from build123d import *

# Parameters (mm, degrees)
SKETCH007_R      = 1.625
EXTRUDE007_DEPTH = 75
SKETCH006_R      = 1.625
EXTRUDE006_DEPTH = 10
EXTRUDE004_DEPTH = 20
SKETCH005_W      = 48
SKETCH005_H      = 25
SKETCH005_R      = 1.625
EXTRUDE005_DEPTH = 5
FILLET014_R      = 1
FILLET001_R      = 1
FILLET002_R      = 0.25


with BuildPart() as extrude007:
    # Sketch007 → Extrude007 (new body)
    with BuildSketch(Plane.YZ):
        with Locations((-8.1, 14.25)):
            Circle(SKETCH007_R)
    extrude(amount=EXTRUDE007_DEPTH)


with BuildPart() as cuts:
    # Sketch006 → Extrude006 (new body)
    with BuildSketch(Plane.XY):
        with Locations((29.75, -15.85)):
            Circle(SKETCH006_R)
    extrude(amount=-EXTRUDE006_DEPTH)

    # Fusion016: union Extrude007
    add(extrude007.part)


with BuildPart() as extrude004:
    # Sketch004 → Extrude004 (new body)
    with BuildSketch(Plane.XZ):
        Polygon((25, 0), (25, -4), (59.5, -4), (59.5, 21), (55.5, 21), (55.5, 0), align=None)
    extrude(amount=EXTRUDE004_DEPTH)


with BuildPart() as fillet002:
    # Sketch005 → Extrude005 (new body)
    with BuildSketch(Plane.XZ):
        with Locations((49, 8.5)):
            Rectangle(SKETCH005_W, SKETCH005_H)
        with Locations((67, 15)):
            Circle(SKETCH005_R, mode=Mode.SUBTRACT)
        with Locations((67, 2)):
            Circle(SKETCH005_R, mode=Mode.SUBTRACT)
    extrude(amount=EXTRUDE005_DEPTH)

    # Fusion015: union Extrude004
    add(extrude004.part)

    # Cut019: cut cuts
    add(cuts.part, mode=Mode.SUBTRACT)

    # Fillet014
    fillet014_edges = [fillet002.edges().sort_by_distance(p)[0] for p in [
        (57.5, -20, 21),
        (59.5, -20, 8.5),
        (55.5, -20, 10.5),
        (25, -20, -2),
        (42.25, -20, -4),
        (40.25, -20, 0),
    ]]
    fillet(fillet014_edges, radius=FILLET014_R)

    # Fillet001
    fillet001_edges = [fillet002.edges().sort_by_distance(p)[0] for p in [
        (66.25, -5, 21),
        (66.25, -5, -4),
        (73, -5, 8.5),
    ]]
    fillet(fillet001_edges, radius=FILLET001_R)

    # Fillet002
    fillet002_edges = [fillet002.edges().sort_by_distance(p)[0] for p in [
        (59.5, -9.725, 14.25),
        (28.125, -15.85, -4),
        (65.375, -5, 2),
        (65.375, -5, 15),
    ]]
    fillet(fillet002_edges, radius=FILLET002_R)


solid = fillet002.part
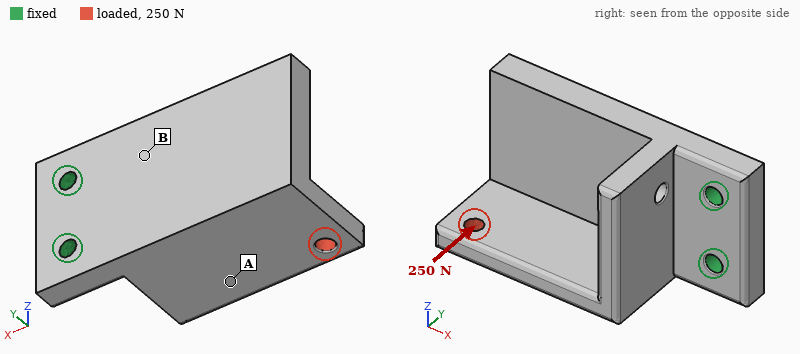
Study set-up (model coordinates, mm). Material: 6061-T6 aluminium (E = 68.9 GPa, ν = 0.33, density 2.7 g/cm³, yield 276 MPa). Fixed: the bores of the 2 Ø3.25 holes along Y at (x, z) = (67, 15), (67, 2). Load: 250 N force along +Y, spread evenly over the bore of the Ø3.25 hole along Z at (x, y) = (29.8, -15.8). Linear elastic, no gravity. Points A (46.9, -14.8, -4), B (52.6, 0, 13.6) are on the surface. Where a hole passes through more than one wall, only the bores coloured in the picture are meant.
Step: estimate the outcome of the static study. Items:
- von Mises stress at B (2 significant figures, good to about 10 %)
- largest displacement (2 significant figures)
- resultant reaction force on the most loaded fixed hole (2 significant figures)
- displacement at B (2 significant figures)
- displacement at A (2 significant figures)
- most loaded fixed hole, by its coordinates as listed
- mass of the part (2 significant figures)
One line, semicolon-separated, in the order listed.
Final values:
30 MPa; 0.24 mm; 270 N; 0.041 mm; 0.11 mm; (67, 2); 25 g
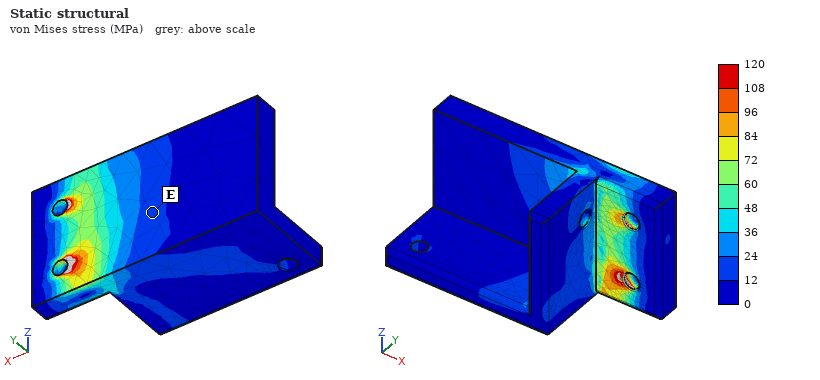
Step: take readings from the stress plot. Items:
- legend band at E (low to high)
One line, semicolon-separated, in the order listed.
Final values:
12 to 24 MPa
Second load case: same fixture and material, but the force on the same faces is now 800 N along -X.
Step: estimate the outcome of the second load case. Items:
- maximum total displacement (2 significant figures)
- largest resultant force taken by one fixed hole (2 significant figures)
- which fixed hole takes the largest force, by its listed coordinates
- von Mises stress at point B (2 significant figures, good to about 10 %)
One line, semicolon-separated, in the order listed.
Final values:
0.31 mm; 960 N; (67, 2); 41 MPa
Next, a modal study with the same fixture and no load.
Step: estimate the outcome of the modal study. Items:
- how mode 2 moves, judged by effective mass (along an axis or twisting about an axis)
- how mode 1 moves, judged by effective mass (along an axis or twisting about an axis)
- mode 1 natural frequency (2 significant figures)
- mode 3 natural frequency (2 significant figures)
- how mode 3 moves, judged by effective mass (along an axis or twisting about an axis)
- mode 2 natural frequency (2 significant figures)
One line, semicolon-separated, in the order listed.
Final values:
along Z; along Y; 2000 Hz; 7500 Hz; along Z; 5700 Hz
